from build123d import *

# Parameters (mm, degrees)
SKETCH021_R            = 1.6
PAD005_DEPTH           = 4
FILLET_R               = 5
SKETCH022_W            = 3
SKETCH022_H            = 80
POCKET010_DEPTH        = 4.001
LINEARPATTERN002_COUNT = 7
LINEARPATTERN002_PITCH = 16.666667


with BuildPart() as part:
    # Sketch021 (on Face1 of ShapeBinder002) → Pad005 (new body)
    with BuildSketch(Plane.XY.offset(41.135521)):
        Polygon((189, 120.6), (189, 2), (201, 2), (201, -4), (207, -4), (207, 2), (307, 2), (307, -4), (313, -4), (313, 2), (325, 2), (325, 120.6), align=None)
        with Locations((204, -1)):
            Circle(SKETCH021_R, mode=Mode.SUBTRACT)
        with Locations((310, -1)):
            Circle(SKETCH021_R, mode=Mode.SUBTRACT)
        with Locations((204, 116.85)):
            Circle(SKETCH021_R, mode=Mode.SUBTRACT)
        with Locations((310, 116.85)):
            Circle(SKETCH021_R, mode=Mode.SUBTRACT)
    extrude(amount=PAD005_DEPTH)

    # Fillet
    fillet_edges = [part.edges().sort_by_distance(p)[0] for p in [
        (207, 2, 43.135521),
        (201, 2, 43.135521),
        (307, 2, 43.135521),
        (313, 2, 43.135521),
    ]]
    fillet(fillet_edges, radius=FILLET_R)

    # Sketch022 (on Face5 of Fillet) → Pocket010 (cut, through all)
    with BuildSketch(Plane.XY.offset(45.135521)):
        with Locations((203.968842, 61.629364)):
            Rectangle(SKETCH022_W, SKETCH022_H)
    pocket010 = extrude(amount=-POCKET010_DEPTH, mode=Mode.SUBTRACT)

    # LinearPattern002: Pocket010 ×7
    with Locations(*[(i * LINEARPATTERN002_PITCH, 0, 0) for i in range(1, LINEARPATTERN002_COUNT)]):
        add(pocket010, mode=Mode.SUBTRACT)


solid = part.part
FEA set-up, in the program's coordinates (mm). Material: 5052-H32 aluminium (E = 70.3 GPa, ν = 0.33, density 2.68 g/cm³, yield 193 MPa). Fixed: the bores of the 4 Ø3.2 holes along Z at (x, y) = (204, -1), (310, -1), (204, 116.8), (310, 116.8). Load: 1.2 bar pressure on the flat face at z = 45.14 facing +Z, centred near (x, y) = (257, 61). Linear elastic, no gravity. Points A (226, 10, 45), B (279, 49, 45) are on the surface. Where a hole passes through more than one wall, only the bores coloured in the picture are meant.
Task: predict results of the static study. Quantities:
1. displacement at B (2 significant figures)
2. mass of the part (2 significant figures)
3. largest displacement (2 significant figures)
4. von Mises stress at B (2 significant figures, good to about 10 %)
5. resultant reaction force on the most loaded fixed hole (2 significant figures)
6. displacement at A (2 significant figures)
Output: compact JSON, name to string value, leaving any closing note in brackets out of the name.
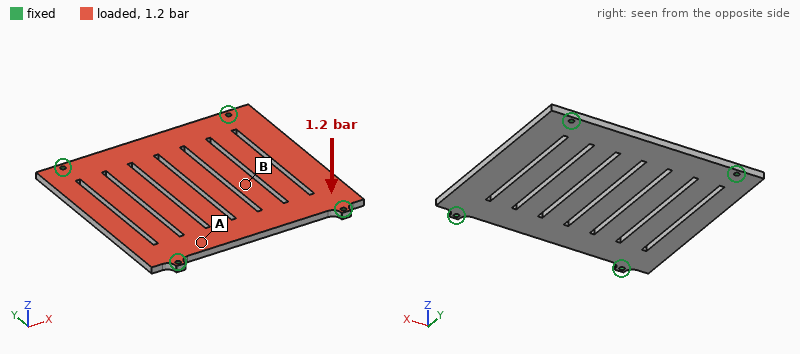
{"displacement at B": "0.57 mm", "mass of the part": "160 g", "largest displacement": "0.70 mm", "von Mises stress at B": "43 MPa", "resultant reaction force on the most loaded fixed hole": "470 N", "displacement at A": "0.24 mm"}
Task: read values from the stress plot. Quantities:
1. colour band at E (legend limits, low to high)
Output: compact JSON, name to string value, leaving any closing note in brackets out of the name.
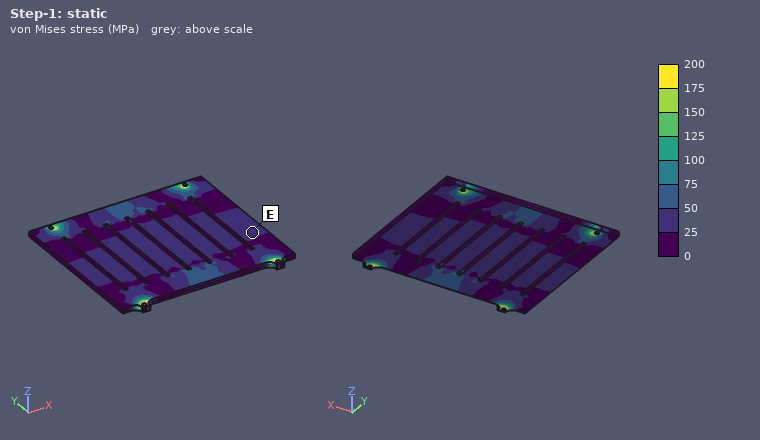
{"colour band at E": "25 to 50 MPa"}
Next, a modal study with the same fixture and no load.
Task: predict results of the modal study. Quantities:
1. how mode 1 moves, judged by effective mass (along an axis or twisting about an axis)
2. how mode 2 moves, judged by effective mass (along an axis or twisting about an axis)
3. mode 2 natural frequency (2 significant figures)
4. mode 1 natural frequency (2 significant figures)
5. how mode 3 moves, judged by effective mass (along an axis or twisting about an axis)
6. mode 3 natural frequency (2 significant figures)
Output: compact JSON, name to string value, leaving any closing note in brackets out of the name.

{"how mode 1 moves, judged by effective mass": "along Z", "how mode 2 moves, judged by effective mass": "twisting about Y", "mode 2 natural frequency": "1300 Hz", "mode 1 natural frequency": "790 Hz", "how mode 3 moves, judged by effective mass": "along Z", "mode 3 natural frequency": "1400 Hz"}
